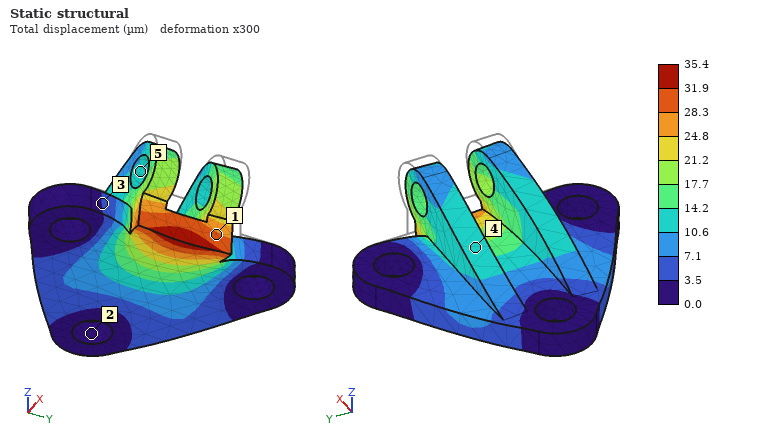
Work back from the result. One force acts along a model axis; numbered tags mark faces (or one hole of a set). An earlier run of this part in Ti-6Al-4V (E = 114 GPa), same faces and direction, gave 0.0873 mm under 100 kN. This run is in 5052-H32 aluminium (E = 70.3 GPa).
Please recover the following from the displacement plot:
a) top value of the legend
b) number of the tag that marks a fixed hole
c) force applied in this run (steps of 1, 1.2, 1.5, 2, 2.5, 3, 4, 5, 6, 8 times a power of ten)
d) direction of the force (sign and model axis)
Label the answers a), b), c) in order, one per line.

a) 35.4 µm
b) 2
c) 25 kN
d) -X
